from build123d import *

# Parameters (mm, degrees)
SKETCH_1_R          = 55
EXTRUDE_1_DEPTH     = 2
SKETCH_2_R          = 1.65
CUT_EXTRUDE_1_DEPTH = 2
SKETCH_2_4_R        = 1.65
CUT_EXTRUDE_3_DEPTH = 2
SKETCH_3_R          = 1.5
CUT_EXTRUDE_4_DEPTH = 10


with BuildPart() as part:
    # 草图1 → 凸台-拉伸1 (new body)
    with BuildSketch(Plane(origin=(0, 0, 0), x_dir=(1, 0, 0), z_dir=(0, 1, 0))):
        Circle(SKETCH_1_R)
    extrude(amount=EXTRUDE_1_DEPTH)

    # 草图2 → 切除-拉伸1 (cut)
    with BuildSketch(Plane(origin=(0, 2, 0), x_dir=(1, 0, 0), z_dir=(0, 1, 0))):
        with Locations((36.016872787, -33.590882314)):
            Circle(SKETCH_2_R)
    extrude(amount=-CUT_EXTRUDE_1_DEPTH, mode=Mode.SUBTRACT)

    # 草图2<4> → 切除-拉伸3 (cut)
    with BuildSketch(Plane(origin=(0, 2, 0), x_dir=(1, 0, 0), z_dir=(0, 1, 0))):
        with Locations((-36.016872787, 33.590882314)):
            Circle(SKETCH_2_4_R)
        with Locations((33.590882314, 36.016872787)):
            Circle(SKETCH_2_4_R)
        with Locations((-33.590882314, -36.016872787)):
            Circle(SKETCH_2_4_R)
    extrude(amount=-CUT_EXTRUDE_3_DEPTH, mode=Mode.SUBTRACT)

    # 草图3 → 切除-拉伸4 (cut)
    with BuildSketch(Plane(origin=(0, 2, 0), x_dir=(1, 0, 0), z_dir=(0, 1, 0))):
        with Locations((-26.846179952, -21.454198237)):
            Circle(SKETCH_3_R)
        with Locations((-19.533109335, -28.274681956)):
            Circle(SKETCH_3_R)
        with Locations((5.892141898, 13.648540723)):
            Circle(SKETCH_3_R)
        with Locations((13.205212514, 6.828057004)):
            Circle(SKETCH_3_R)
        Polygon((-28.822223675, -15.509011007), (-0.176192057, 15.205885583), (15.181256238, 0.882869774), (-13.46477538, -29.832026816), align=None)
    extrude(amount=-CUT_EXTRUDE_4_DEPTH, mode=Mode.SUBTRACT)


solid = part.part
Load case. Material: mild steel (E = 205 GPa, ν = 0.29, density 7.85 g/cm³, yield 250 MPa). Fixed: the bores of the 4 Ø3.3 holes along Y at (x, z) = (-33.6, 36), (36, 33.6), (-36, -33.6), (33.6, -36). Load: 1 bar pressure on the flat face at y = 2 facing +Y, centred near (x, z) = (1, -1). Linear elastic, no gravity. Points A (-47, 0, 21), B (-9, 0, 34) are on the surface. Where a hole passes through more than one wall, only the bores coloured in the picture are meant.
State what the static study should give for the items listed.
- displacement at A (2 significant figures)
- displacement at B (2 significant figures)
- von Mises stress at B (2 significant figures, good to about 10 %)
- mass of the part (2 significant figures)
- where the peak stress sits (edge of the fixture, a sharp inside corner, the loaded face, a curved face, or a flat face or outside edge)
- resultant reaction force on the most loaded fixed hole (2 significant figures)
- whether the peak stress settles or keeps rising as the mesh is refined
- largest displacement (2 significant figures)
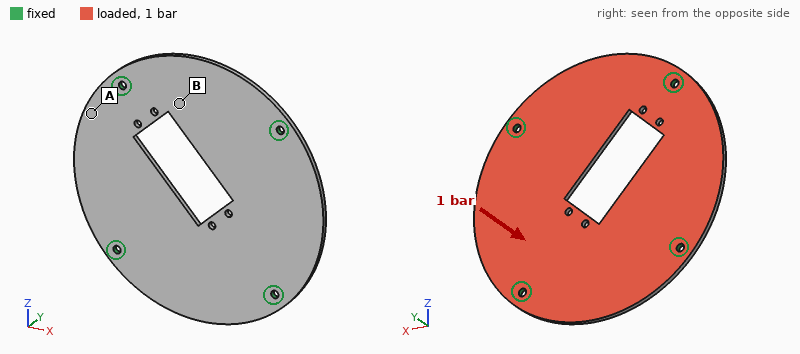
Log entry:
0.028 mm
0.055 mm
38 MPa
130 g
edge of the fixture
220 N
keeps rising
0.11 mm
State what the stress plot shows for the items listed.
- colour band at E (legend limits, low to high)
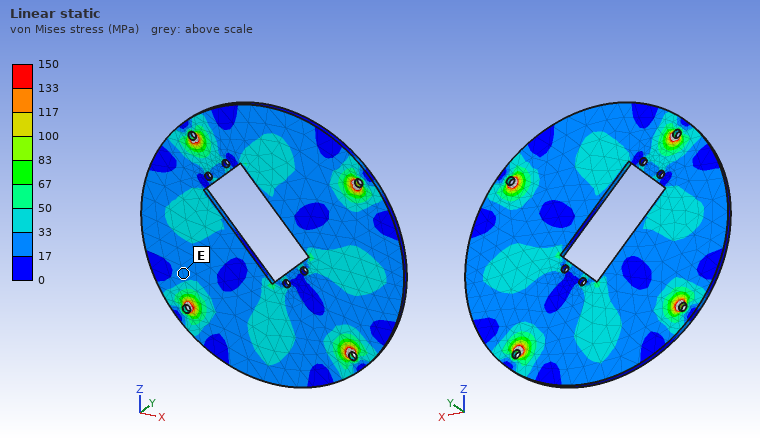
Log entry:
17 to 33 MPa
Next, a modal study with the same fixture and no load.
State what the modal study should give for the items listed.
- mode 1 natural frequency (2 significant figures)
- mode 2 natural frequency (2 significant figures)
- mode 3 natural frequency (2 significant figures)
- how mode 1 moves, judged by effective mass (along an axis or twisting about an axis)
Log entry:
1600 Hz
1700 Hz
1800 Hz
along Y
